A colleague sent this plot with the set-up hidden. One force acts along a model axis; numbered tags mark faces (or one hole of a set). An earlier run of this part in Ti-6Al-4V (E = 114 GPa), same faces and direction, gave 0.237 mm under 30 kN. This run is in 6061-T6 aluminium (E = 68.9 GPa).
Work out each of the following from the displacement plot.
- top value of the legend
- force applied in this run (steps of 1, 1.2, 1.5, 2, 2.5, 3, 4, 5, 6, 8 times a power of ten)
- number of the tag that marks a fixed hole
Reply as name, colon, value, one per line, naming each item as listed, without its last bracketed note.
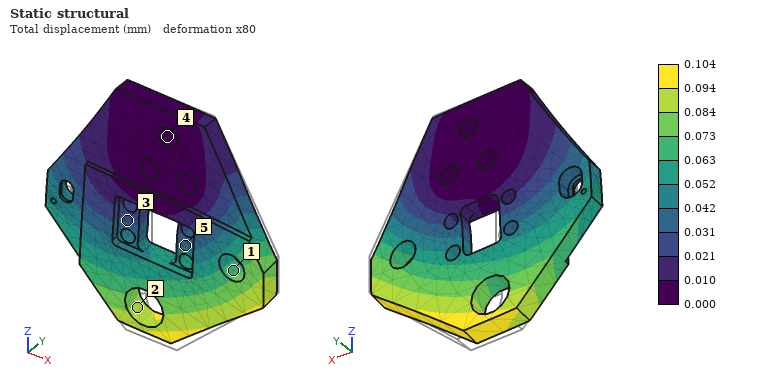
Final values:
top value of the legend: 0.104 mm
force applied in this run: 8 kN
number of the tag that marks a fixed hole: 4
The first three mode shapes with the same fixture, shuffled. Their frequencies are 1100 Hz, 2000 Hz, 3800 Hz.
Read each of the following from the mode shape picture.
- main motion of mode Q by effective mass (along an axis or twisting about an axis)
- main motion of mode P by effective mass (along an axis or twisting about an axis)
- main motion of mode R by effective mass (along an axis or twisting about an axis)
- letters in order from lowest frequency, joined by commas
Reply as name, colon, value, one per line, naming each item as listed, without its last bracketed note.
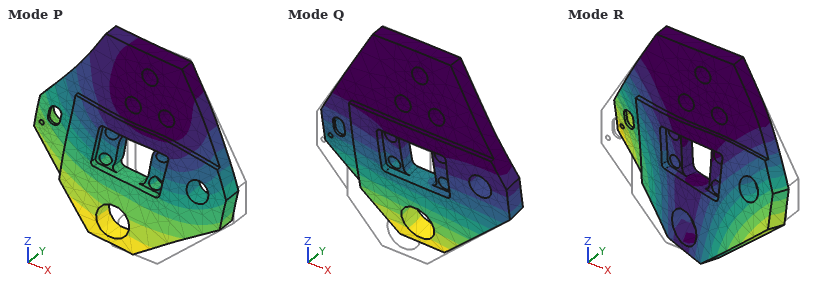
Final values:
main motion of mode Q by effective mass: along Y
main motion of mode P by effective mass: along X
main motion of mode R by effective mass: twisting about Z
letters in order from lowest frequency, joined by commas: Q, R, P
